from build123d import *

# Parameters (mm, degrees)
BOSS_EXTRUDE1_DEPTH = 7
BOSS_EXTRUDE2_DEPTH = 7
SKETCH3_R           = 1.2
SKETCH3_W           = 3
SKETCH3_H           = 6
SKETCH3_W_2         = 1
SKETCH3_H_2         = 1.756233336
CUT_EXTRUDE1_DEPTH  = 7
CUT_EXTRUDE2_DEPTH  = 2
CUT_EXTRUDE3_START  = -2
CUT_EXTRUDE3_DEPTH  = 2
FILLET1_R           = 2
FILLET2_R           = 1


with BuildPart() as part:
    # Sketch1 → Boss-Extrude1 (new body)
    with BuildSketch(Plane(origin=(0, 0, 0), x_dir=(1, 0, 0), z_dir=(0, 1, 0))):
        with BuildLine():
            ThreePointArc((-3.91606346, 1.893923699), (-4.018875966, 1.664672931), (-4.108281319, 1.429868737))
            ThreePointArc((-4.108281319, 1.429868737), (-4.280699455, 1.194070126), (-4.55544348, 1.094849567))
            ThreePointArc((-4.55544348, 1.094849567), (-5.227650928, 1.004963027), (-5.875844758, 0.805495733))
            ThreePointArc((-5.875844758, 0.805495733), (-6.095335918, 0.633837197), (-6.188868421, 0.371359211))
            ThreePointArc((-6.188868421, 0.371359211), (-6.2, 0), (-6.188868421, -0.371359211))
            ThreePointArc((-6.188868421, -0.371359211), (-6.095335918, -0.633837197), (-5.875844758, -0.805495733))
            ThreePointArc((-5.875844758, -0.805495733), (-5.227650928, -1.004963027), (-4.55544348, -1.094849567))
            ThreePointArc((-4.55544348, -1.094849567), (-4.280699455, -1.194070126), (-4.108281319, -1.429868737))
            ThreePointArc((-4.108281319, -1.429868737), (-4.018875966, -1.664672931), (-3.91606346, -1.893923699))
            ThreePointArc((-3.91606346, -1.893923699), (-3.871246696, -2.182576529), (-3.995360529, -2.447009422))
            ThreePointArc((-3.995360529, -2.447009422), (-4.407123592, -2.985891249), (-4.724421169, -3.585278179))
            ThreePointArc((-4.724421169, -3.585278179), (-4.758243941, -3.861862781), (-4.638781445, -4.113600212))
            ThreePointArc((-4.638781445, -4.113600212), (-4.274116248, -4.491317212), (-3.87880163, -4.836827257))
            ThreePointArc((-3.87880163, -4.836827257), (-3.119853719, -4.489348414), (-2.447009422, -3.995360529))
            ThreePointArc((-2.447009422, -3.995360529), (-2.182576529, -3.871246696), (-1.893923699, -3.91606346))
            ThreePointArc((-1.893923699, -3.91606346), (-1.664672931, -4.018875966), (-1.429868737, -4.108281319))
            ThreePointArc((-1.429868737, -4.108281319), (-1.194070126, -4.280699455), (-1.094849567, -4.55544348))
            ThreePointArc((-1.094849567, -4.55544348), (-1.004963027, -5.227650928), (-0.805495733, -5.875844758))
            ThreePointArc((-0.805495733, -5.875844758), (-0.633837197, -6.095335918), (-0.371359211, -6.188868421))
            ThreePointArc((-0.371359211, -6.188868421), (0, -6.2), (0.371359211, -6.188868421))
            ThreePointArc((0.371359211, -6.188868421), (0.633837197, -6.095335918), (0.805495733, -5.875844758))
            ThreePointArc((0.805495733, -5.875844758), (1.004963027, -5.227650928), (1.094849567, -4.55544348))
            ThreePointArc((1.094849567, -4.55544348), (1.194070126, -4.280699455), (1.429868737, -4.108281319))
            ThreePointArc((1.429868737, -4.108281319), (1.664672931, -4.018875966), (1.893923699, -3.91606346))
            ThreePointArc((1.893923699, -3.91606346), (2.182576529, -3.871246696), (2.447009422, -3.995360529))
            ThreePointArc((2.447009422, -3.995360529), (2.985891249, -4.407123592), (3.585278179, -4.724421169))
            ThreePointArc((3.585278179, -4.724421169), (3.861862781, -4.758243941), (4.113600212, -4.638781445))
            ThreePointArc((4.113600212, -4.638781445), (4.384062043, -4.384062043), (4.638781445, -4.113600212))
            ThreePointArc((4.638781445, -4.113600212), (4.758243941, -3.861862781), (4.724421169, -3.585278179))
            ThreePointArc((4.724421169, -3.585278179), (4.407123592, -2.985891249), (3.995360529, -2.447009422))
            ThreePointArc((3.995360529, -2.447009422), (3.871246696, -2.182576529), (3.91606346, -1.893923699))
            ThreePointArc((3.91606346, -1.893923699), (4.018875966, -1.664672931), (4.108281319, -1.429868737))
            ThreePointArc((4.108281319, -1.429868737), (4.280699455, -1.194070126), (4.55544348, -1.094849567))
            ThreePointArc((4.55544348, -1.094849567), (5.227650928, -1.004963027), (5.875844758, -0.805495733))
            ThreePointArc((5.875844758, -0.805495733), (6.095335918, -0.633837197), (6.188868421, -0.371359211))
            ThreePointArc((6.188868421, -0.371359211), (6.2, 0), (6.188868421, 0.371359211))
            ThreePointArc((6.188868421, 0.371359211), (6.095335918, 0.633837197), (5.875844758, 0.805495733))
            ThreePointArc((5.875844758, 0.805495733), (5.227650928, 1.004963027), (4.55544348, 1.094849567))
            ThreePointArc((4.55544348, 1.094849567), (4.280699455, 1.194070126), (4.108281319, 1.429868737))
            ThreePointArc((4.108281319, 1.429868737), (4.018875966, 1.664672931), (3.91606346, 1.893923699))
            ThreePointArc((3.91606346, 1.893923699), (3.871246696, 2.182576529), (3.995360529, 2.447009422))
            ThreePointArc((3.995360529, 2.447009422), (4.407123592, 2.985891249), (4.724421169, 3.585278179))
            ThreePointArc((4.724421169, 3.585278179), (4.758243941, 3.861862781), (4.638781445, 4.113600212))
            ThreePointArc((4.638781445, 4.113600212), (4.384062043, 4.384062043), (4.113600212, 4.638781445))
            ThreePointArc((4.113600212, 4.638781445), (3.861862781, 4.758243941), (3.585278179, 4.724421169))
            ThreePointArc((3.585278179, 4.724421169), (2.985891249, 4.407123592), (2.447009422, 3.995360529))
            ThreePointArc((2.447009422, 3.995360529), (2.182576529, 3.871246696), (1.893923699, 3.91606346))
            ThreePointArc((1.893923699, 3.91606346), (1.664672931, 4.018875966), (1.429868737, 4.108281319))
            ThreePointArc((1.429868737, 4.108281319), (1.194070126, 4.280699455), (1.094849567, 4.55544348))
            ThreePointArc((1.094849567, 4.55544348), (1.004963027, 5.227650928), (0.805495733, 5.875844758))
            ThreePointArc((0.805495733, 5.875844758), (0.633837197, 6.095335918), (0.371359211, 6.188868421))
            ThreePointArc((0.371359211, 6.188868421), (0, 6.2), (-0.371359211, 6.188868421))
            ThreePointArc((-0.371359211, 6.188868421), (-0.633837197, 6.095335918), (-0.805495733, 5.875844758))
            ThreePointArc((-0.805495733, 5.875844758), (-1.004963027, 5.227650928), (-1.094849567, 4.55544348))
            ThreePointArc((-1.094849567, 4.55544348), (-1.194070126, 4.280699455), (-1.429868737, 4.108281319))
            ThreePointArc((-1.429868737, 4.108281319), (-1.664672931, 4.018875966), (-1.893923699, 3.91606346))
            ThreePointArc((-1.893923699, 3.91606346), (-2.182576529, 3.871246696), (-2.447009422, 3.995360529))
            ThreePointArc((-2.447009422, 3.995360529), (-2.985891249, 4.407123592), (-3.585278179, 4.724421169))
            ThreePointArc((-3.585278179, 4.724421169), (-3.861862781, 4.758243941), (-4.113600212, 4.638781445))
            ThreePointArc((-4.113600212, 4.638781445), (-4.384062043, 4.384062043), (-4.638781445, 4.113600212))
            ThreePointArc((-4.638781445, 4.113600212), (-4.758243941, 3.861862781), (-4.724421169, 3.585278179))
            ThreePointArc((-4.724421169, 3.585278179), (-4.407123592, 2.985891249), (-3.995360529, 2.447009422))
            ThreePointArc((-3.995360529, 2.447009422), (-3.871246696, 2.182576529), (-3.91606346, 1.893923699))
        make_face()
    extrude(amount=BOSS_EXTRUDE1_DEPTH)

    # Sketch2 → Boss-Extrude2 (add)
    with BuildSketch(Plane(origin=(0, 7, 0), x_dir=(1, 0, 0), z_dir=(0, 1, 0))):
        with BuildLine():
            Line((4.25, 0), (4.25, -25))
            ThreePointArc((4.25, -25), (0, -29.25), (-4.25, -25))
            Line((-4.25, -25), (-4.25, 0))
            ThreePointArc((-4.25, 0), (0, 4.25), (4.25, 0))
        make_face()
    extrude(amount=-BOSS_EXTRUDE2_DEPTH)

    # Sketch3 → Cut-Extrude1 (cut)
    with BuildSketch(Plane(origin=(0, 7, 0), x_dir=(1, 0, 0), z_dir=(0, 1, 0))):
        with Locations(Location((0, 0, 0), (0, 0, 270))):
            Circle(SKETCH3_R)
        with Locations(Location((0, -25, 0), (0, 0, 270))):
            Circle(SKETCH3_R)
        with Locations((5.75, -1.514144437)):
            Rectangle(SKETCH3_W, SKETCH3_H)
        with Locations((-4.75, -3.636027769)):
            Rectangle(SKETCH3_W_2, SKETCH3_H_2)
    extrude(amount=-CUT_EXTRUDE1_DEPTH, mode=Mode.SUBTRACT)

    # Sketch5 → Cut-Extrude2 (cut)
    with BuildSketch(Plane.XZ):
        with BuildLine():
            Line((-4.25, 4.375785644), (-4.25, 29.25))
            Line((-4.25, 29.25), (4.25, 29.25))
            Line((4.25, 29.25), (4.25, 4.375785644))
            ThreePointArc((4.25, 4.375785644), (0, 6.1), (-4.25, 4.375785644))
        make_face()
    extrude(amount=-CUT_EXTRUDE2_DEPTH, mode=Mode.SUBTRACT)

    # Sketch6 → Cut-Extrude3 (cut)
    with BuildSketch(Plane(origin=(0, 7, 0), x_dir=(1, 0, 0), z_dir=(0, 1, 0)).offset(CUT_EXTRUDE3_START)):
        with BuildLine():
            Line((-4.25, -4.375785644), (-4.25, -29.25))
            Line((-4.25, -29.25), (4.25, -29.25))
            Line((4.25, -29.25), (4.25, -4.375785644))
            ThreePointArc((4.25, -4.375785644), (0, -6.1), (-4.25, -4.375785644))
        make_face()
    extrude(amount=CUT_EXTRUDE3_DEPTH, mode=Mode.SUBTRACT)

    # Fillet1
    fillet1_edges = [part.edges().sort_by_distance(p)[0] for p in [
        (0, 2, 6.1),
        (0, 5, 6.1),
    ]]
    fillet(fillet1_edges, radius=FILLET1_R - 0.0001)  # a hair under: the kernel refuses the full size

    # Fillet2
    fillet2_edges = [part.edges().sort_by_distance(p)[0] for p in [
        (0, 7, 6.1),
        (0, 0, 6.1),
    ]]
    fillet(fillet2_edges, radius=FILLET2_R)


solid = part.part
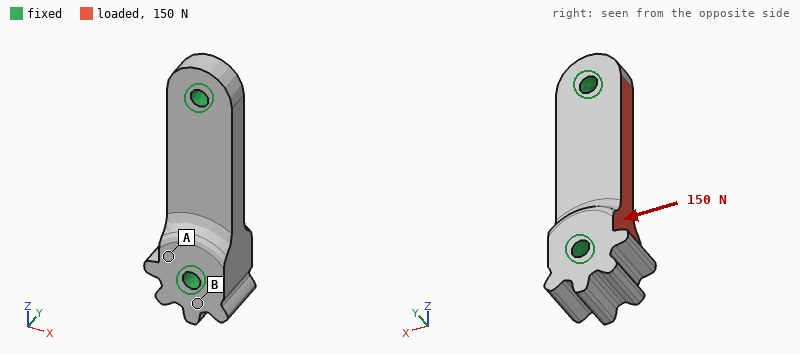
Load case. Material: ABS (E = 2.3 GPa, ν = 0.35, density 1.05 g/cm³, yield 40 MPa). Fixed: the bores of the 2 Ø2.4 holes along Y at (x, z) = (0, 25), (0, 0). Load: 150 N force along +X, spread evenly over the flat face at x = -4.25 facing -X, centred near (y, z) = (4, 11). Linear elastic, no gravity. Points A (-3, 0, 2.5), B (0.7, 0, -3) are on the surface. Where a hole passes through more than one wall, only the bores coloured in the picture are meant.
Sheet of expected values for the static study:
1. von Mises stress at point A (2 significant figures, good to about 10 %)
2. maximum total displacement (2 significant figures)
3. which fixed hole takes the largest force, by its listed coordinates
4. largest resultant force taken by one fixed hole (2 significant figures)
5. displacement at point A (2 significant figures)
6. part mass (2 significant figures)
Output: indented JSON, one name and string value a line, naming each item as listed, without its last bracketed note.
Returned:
{
  "von Mises stress at point A": "2.7 MPa",
  "maximum total displacement": "44 µm",
  "which fixed hole takes the largest force, by its listed coordinates": "(0, 0)",
  "largest resultant force taken by one fixed hole": "88 N",
  "displacement at point A": "13 µm",
  "part mass": "1.2 g"
}
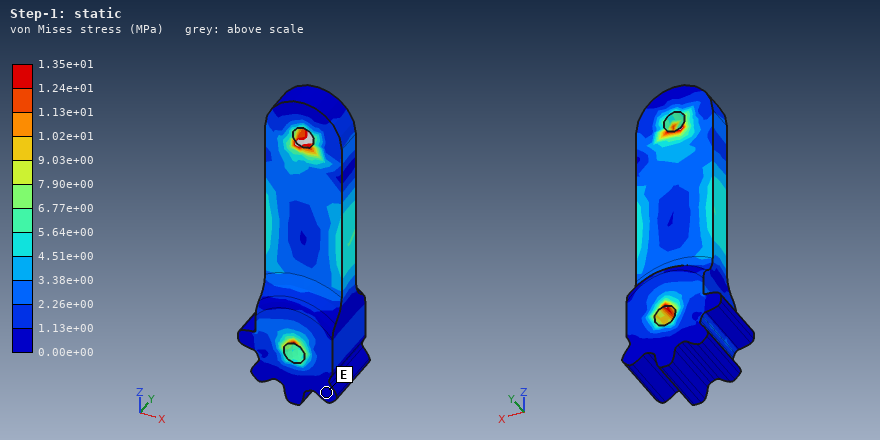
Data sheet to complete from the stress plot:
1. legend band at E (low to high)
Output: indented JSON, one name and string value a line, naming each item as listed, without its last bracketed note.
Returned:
{
  "legend band at E": "0.00e+00 to 1.13e+00 MPa"
}
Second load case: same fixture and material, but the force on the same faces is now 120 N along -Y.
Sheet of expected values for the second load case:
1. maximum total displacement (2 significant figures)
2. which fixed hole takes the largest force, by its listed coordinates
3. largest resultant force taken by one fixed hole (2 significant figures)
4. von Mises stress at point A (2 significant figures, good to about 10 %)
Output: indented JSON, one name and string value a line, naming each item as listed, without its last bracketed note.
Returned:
{
  "maximum total displacement": "0.13 mm",
  "which fixed hole takes the largest force, by its listed coordinates": "(0, 0)",
  "largest resultant force taken by one fixed hole": "77 N",
  "von Mises stress at point A": "5.5 MPa"
}
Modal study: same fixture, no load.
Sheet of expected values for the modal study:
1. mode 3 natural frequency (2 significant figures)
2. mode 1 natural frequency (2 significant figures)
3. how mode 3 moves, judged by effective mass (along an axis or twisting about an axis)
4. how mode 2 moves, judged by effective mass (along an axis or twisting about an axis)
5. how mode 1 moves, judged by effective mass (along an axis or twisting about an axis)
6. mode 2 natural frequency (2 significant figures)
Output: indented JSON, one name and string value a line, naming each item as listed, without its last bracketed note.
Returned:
{
  "mode 3 natural frequency": "15 kHz",
  "mode 1 natural frequency": "9800 Hz",
  "how mode 3 moves, judged by effective mass": "twisting about Z",
  "how mode 2 moves, judged by effective mass": "along X",
  "how mode 1 moves, judged by effective mass": "along Y",
  "mode 2 natural frequency": "12 kHz"
}
